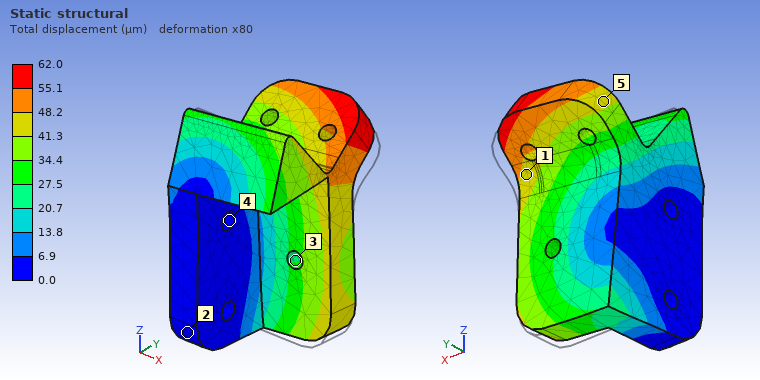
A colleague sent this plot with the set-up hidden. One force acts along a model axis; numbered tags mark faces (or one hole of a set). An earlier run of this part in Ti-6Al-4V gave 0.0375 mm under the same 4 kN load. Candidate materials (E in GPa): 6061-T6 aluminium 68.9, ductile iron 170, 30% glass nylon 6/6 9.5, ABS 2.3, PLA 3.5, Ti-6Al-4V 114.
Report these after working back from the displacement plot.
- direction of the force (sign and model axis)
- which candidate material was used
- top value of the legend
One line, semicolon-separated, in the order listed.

+Z; 6061-T6 aluminium; 62.0 µm
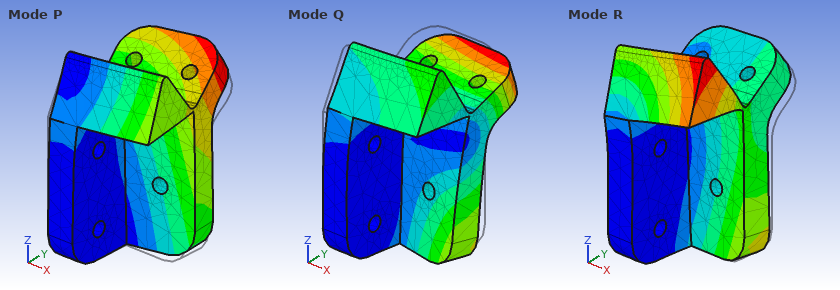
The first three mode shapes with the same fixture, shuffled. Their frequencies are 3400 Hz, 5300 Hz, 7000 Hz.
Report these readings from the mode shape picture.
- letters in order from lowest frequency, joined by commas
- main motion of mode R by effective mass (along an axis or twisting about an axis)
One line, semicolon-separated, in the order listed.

P, R, Q; along Z
